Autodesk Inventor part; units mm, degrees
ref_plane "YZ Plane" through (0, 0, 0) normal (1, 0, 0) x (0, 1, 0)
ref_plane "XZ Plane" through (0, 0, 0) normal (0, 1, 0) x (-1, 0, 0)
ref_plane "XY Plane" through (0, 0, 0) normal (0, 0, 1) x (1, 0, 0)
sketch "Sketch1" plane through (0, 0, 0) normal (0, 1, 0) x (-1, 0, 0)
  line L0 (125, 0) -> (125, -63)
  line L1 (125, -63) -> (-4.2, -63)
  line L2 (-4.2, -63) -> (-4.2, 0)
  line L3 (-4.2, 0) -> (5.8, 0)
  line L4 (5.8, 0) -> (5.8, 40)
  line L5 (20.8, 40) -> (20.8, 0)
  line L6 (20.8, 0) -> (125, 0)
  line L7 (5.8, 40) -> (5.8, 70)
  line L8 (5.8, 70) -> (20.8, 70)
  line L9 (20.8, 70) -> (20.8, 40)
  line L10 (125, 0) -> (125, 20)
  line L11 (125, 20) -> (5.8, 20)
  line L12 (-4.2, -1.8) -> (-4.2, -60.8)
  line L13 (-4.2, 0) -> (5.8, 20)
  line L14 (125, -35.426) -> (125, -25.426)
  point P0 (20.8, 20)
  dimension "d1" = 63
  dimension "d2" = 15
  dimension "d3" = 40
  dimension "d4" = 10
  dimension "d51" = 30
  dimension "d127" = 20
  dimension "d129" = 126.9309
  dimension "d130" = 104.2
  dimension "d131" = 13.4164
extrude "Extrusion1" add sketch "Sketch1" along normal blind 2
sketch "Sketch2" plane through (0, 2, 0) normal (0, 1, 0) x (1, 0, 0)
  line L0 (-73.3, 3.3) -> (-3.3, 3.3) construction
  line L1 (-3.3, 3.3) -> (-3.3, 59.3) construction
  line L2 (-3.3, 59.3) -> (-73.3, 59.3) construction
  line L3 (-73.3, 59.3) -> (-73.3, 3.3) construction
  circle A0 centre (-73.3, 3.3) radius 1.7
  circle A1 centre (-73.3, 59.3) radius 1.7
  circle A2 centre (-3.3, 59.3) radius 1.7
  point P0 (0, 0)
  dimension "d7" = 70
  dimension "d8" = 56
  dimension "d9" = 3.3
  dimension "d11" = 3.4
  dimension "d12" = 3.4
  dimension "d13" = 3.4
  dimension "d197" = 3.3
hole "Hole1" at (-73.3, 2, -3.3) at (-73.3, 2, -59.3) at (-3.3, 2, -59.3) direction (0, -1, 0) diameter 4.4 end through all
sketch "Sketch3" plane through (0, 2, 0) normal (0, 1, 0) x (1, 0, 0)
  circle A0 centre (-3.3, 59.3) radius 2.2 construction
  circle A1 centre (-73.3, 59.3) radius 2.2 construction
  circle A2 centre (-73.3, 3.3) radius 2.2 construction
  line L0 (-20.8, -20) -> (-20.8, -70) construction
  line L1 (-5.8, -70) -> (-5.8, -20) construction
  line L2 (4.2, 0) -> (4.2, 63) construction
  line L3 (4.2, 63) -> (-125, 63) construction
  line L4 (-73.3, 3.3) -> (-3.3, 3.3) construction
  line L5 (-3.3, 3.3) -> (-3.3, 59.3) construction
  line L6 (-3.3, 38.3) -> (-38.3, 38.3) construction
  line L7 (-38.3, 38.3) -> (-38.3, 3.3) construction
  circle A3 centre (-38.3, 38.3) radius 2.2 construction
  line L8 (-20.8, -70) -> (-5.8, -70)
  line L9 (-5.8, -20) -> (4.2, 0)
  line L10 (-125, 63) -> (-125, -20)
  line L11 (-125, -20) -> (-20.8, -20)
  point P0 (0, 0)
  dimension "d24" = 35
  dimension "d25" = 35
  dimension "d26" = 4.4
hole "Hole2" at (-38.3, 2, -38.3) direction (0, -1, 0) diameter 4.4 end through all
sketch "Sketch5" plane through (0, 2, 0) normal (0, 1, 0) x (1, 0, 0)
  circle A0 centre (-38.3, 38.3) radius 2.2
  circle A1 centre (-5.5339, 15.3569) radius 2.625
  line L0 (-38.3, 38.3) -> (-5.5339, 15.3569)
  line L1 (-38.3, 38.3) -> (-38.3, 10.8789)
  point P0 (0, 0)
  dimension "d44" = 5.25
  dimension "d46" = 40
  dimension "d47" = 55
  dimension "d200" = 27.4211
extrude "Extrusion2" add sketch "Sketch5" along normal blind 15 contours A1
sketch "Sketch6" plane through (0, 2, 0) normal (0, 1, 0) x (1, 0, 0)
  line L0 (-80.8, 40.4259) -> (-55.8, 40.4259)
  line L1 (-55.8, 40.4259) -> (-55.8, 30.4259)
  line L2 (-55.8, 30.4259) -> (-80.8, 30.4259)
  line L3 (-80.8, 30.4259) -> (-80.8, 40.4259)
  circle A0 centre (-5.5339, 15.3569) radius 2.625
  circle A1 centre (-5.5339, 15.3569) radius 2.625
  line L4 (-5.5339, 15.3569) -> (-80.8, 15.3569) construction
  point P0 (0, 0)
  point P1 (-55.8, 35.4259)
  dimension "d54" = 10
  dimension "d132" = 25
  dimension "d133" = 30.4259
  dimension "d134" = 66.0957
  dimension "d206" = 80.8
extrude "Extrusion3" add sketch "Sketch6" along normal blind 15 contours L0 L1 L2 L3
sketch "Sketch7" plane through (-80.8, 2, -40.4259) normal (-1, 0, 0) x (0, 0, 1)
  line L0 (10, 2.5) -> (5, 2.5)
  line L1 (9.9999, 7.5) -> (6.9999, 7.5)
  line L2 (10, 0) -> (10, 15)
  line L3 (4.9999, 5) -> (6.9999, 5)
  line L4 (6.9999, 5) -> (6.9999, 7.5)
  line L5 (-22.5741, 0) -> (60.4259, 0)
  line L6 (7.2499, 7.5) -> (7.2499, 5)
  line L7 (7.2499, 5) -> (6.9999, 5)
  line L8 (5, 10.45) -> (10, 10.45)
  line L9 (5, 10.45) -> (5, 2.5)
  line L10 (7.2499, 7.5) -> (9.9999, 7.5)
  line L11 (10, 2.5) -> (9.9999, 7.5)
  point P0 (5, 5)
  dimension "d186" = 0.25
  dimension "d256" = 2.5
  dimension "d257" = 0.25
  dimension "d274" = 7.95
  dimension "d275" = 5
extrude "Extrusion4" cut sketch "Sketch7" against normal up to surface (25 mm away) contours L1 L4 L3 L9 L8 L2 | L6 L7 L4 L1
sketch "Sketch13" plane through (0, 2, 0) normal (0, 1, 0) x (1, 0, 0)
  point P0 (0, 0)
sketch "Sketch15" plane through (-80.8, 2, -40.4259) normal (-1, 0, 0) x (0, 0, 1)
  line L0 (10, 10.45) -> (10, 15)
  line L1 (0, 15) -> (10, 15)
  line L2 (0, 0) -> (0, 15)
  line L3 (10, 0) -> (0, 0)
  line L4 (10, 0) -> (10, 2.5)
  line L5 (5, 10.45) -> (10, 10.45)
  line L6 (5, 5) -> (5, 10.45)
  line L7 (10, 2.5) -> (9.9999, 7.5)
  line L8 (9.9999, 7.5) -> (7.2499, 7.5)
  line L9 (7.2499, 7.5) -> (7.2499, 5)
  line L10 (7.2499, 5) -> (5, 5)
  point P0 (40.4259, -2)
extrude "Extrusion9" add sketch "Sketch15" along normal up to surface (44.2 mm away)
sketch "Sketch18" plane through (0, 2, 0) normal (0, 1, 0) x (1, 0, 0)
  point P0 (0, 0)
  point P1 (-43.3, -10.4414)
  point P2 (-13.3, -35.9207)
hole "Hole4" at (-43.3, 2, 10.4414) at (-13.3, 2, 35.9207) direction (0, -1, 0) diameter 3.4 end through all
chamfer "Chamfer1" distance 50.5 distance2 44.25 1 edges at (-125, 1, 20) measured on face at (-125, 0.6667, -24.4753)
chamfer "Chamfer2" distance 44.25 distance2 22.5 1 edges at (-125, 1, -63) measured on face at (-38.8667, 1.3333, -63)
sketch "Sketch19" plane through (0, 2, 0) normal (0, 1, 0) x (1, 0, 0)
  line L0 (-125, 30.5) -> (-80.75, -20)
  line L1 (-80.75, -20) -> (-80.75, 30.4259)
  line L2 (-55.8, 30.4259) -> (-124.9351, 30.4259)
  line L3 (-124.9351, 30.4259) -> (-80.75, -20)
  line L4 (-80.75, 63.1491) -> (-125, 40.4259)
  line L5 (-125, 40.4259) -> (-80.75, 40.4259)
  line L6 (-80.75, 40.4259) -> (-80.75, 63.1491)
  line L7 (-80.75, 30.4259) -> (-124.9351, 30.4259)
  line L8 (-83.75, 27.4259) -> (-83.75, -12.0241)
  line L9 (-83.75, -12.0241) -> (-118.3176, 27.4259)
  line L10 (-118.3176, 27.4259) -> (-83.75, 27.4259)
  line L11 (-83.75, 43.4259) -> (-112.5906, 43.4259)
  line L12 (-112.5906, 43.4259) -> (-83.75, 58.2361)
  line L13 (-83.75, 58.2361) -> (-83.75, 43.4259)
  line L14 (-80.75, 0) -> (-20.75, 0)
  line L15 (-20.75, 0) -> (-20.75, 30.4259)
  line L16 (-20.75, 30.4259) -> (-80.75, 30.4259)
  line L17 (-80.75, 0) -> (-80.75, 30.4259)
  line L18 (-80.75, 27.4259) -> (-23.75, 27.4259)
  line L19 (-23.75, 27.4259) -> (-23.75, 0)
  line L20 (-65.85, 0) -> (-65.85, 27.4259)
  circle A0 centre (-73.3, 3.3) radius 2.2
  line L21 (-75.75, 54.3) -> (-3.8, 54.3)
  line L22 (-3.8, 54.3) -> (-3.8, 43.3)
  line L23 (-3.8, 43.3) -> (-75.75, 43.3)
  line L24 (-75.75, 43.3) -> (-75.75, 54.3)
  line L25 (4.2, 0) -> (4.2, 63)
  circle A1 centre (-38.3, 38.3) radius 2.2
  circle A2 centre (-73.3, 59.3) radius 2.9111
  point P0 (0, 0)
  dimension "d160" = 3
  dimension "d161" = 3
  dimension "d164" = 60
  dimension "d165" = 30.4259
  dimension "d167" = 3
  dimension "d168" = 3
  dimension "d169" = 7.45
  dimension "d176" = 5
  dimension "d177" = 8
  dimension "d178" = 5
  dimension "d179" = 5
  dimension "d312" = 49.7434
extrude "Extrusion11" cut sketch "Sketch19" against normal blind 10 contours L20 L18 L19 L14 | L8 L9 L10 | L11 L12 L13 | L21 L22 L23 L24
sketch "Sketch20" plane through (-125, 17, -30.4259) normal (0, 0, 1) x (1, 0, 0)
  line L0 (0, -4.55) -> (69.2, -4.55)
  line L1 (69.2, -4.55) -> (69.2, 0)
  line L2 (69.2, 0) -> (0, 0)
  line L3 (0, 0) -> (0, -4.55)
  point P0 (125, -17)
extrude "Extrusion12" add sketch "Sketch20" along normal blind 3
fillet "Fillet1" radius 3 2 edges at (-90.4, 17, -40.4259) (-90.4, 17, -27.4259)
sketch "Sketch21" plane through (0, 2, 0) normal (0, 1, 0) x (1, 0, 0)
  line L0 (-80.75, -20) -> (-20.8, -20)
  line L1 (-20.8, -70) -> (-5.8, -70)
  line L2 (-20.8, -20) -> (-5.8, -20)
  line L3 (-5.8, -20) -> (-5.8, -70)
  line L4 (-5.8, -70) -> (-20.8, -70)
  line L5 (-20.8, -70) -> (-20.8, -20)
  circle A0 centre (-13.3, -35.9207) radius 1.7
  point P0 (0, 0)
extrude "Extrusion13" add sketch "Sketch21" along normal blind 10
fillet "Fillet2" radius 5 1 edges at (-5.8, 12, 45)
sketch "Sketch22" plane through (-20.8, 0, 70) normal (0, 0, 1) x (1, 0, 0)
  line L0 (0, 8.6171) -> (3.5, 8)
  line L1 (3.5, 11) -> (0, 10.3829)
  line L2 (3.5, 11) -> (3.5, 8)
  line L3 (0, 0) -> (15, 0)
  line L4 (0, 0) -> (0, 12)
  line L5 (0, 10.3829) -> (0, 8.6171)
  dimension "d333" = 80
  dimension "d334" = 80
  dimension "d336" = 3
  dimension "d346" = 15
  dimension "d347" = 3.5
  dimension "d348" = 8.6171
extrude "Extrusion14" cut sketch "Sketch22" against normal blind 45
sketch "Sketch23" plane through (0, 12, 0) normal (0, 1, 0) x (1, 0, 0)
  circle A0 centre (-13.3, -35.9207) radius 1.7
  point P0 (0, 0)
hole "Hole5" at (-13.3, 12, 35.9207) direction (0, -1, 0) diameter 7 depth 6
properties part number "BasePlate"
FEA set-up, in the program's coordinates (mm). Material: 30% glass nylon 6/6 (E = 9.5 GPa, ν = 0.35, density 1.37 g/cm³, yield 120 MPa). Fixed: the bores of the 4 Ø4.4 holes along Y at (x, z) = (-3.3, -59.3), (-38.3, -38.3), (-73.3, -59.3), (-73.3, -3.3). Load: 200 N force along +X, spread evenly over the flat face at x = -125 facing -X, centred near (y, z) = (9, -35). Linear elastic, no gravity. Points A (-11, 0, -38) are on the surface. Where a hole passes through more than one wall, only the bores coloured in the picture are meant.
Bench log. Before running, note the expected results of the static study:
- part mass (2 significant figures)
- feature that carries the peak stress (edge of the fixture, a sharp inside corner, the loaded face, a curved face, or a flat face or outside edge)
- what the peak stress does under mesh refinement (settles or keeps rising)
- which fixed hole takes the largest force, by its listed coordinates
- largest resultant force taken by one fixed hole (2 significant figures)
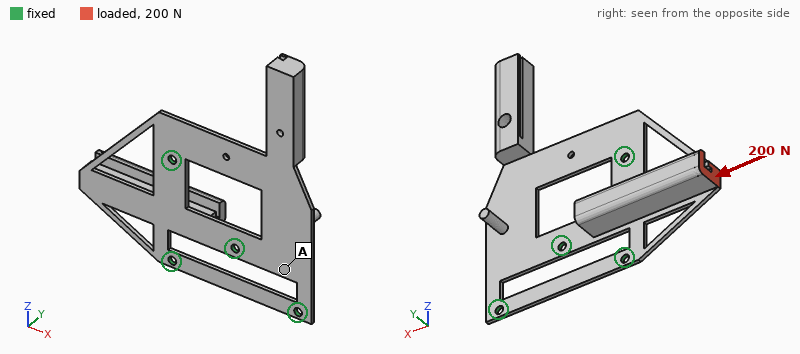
41 g
edge of the fixture
keeps rising
(-38.3, -38.3)
150 N
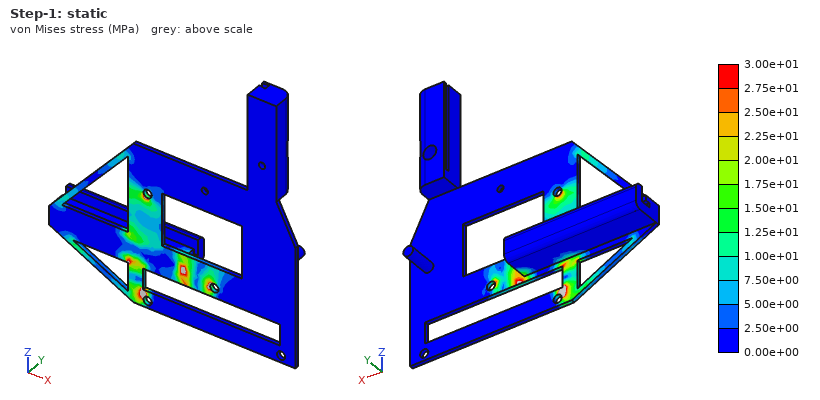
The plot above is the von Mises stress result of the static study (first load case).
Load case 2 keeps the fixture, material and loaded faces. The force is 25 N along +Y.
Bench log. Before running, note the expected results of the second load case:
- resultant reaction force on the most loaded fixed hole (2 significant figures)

37 N
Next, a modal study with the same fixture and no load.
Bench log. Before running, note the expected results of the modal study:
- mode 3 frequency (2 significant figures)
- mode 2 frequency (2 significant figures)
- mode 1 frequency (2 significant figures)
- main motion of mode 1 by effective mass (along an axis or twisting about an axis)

310 Hz
310 Hz
57 Hz
along Y
